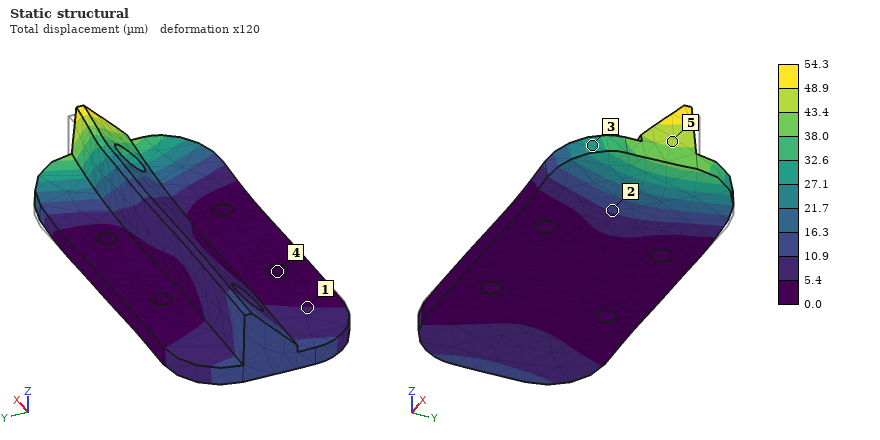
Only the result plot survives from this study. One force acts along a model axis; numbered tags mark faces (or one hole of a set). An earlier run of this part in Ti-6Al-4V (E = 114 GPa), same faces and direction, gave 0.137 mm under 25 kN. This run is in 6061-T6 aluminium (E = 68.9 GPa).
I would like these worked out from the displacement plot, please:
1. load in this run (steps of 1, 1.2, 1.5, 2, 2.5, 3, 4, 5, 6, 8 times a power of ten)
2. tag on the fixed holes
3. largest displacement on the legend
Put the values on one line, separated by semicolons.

6 kN; 4; 54.3 µm
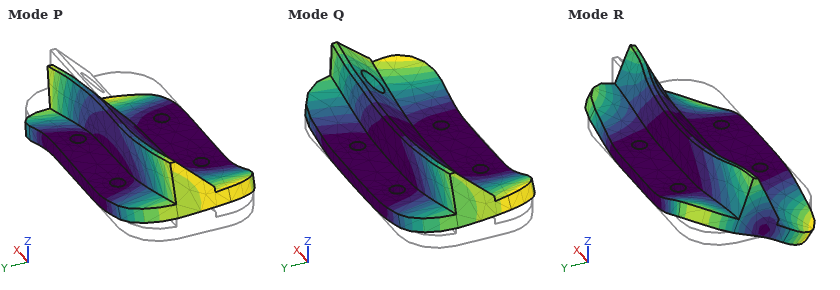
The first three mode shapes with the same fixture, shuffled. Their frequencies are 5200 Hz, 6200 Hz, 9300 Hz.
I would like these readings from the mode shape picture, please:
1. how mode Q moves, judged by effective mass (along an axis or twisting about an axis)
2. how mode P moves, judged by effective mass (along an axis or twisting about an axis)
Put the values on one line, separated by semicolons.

along Z; twisting about Y
